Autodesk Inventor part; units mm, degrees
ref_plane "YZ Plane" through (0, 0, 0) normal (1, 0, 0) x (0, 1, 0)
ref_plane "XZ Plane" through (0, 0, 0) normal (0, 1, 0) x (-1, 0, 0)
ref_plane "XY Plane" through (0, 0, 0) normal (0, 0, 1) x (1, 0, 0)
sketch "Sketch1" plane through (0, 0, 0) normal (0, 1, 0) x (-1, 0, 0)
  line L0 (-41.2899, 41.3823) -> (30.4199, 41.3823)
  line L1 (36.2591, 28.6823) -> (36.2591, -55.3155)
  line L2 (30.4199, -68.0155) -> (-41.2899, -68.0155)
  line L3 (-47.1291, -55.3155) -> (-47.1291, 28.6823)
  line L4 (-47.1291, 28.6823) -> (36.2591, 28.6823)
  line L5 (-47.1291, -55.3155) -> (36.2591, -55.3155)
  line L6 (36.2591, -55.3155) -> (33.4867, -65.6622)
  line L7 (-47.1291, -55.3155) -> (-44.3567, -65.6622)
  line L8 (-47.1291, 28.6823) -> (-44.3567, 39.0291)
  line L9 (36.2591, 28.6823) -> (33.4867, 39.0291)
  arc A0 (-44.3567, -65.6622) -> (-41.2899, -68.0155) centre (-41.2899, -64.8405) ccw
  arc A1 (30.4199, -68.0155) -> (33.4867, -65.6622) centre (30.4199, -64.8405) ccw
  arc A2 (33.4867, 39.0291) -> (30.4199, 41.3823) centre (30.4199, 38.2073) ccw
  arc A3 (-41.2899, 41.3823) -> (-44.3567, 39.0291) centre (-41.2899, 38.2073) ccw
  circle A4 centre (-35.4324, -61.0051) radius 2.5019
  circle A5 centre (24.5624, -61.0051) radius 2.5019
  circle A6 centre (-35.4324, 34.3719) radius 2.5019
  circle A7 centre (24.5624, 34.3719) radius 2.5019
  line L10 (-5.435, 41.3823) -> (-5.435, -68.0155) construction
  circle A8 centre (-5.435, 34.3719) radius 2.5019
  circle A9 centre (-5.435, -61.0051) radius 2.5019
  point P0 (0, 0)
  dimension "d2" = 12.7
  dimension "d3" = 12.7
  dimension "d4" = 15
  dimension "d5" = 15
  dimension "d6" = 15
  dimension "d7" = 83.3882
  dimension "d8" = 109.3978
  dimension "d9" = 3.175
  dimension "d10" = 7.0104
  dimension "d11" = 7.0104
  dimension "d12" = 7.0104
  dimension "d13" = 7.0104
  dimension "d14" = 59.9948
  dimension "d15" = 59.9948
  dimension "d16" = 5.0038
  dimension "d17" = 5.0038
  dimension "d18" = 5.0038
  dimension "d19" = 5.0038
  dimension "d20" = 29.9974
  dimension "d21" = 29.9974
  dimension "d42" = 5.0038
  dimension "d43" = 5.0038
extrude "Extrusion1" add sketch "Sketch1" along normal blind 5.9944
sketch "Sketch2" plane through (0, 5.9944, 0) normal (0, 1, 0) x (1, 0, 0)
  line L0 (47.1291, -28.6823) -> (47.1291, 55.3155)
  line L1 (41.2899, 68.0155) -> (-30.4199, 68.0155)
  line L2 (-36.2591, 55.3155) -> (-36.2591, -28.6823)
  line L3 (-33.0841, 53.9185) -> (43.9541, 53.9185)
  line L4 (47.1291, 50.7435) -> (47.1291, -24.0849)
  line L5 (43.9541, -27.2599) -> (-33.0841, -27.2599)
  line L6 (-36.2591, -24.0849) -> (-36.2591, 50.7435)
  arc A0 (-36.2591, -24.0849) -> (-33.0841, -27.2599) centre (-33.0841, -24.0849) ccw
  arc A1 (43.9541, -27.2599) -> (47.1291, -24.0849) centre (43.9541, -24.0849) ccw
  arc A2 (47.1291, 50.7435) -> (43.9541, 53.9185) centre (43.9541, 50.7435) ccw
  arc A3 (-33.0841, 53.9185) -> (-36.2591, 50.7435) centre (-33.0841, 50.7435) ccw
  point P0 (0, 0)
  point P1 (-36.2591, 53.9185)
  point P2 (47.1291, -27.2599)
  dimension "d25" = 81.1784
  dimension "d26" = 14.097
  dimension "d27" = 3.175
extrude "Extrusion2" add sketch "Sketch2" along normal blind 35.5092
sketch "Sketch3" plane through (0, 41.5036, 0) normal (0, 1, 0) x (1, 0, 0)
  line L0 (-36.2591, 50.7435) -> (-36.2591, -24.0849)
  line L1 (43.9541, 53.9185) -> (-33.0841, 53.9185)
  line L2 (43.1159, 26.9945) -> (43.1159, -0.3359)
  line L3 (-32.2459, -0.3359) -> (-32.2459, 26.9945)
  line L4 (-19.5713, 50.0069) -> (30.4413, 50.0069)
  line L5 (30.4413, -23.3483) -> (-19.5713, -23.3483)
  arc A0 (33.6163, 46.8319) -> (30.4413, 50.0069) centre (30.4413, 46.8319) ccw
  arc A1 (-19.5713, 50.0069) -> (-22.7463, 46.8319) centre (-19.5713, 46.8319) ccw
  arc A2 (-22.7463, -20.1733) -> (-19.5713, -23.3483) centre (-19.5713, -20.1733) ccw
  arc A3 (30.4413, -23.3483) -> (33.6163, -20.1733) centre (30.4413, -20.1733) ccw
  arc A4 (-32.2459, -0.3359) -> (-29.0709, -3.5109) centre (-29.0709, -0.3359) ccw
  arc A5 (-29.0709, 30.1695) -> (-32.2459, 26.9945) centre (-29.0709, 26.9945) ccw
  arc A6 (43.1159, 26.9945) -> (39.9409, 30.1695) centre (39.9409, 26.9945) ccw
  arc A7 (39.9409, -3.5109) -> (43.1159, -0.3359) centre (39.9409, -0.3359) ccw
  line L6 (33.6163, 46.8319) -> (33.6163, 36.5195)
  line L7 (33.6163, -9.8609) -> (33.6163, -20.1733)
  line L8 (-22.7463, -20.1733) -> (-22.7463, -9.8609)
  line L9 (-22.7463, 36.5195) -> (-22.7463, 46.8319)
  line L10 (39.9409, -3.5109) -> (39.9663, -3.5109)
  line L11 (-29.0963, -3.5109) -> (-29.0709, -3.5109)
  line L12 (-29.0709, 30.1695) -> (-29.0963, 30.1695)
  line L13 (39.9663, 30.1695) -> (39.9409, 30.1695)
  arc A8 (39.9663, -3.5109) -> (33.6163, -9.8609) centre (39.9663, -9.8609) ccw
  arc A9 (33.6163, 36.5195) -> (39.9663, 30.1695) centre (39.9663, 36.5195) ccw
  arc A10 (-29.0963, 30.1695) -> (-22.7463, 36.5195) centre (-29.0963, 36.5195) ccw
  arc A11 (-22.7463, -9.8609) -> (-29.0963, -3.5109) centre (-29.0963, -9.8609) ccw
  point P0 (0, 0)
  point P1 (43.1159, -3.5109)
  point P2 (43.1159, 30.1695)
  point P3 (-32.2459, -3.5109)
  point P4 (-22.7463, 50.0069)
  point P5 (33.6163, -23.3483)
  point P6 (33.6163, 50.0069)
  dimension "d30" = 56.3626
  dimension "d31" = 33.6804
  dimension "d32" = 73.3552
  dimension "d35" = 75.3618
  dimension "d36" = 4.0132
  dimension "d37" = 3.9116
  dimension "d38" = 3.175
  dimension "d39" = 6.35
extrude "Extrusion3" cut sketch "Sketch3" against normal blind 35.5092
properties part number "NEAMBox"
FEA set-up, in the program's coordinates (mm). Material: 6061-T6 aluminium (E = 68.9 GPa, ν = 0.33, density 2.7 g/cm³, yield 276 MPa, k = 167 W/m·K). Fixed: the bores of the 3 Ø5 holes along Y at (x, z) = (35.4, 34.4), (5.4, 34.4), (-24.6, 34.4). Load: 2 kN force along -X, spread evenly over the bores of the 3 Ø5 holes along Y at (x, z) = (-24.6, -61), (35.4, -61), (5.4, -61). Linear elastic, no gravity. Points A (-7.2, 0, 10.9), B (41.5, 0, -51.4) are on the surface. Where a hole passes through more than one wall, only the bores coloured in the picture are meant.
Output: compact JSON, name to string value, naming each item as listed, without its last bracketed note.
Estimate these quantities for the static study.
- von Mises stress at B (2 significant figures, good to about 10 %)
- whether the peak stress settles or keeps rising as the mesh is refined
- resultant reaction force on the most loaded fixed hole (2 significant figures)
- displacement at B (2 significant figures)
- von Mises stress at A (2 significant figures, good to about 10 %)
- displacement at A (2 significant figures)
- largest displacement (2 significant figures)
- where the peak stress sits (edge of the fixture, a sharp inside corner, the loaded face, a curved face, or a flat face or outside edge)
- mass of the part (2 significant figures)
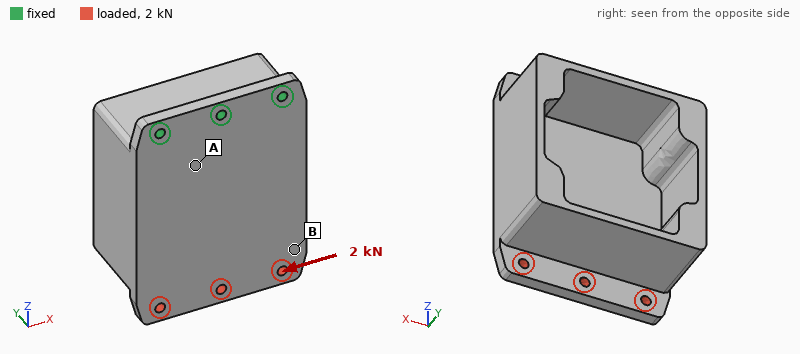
{"von Mises stress at B": "3.9 MPa", "whether the peak stress settles or keeps rising as the mesh is refined": "keeps rising", "resultant reaction force on the most loaded fixed hole": "3.1 kN", "displacement at B": "46 µm", "von Mises stress at A": "13 MPa", "displacement at A": "9.3 µm", "largest displacement": "55 µm", "where the peak stress sits": "edge of the fixture", "mass of the part": "330 g"}
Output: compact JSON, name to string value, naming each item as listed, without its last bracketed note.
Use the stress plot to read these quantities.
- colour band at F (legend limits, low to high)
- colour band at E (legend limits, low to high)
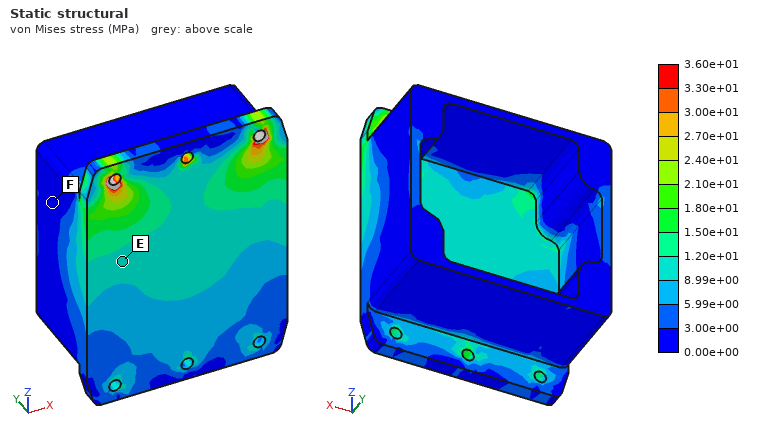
{"colour band at F": "0.00e+00 to 3.00e+00 MPa", "colour band at E": "8.99e+00 to 1.20e+01 MPa"}
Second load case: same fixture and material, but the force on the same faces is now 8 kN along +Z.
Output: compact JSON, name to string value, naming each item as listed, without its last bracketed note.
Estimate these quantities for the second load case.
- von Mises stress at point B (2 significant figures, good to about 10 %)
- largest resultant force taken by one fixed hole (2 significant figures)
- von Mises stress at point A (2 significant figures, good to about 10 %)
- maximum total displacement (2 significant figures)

{"von Mises stress at point B": "21 MPa", "largest resultant force taken by one fixed hole": "2.8 kN", "von Mises stress at point A": "16 MPa", "maximum total displacement": "53 µm"}
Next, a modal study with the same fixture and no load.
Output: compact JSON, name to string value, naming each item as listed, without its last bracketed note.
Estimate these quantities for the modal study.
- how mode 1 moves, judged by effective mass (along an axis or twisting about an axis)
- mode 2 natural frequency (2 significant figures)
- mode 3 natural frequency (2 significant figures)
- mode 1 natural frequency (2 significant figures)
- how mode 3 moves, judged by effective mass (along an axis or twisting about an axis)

{"how mode 1 moves, judged by effective mass": "along Y", "mode 2 natural frequency": "1100 Hz", "mode 3 natural frequency": "2900 Hz", "mode 1 natural frequency": "440 Hz", "how mode 3 moves, judged by effective mass": "along X"}
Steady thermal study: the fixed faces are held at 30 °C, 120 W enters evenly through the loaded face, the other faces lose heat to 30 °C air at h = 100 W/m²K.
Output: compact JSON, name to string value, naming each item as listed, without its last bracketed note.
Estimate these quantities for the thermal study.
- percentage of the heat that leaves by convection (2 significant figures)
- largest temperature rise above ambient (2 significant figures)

{"percentage of the heat that leaves by convection": "69 %", "largest temperature rise above ambient": "59 K"}
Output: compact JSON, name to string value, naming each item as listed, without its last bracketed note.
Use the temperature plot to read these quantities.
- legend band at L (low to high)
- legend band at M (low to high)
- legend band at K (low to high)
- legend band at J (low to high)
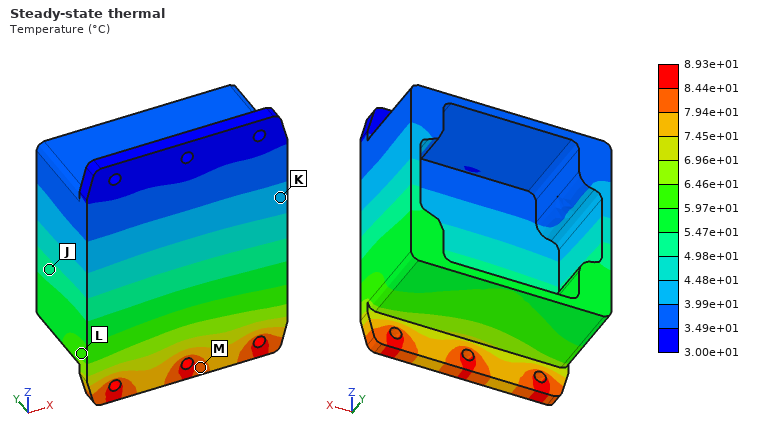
{"legend band at L": "5.97e+01 to 6.46e+01 °C", "legend band at M": "7.94e+01 to 8.44e+01 °C", "legend band at K": "3.99e+01 to 4.48e+01 °C", "legend band at J": "4.98e+01 to 5.47e+01 °C"}
